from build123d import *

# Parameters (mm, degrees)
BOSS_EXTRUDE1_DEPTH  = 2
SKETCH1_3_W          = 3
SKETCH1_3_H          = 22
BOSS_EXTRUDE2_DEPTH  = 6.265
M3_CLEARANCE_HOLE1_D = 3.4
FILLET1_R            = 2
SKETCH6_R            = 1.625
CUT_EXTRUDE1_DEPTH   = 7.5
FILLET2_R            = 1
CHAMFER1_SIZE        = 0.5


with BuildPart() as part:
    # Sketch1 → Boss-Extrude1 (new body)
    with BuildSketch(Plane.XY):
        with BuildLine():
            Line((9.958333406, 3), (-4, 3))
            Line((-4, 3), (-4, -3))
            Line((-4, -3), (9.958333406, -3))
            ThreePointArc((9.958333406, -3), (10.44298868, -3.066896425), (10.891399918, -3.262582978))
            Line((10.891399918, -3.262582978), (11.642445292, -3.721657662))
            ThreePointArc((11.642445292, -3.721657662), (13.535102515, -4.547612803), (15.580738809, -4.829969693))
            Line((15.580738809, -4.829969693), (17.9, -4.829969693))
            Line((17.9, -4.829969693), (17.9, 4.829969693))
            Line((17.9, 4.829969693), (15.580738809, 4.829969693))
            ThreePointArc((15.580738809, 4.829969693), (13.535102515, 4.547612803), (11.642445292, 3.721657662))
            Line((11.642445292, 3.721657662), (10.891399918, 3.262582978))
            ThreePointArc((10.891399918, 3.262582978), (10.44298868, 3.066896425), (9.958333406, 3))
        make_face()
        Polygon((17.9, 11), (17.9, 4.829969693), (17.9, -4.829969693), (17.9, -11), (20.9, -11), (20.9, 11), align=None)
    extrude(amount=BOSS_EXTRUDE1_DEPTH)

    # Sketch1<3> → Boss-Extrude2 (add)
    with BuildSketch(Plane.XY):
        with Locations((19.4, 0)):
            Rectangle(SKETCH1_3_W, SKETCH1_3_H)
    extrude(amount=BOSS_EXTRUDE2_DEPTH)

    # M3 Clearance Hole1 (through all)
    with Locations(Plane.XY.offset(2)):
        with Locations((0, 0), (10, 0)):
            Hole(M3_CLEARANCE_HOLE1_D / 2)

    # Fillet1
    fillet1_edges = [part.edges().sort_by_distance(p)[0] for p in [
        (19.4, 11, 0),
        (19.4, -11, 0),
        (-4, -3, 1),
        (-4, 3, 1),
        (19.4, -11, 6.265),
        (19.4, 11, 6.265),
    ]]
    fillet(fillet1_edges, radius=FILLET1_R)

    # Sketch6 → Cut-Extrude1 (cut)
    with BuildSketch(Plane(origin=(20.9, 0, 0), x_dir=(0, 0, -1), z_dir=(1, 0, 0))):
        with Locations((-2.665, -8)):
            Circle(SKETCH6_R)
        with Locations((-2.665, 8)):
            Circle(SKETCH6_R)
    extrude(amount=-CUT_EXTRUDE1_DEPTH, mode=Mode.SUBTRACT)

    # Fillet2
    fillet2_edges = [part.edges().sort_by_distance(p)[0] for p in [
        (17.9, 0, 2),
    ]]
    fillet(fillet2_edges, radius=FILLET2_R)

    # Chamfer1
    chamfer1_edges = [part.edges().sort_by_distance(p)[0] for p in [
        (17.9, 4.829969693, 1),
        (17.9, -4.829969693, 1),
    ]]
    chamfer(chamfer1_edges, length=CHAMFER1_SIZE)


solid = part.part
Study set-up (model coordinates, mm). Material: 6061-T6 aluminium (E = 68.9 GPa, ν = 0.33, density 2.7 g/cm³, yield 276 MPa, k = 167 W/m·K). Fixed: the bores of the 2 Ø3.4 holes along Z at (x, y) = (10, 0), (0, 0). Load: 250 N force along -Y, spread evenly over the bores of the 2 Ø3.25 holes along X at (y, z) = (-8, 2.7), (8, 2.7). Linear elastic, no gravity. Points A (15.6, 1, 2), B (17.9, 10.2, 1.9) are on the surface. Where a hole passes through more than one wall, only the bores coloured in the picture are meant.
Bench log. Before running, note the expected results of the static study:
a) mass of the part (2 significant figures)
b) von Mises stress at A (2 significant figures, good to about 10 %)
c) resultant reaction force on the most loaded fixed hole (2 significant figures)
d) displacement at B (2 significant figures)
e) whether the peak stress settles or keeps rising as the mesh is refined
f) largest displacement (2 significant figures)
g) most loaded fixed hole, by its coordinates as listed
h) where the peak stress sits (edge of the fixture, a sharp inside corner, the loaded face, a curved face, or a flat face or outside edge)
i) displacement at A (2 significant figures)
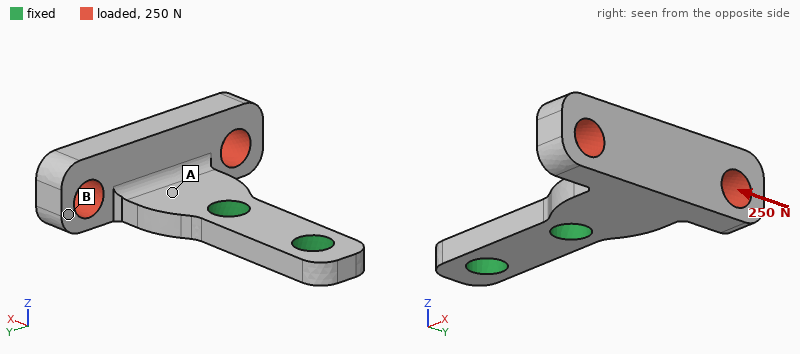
1.7 g
82 MPa
280 N
54 µm
keeps rising
68 µm
(10, 0)
edge of the fixture
16 µm
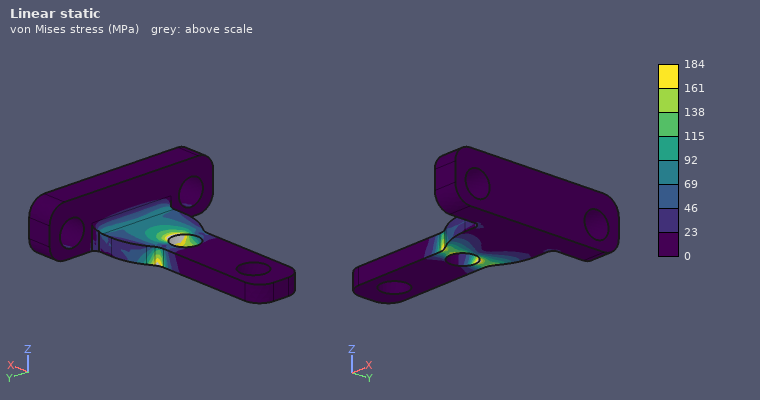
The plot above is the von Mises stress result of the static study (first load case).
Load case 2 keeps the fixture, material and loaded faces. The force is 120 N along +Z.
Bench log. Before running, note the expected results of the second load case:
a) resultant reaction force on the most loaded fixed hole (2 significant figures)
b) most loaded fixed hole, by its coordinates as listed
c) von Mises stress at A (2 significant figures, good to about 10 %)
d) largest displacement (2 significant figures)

120 N
(10, 0)
67 MPa
96 µm
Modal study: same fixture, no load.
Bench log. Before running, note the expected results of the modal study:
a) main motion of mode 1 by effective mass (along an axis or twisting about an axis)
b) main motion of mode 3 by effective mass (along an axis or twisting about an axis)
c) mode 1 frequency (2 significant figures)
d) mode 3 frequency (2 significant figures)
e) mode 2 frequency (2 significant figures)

along Z
along Y
6300 Hz
13 kHz
7600 Hz
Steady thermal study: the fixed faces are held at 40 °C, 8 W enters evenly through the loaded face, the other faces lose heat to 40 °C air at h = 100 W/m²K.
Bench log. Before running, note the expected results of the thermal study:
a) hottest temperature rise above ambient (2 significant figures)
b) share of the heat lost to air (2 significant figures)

28 K
12 %
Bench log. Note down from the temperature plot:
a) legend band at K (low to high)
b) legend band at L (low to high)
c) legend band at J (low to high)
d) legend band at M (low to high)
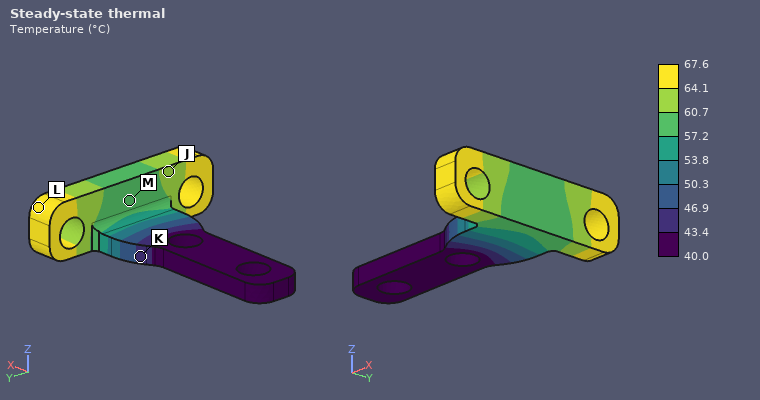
43.4 to 46.9 °C
64.1 to 67.6 °C
60.7 to 64.1 °C
57.2 to 60.7 °C
